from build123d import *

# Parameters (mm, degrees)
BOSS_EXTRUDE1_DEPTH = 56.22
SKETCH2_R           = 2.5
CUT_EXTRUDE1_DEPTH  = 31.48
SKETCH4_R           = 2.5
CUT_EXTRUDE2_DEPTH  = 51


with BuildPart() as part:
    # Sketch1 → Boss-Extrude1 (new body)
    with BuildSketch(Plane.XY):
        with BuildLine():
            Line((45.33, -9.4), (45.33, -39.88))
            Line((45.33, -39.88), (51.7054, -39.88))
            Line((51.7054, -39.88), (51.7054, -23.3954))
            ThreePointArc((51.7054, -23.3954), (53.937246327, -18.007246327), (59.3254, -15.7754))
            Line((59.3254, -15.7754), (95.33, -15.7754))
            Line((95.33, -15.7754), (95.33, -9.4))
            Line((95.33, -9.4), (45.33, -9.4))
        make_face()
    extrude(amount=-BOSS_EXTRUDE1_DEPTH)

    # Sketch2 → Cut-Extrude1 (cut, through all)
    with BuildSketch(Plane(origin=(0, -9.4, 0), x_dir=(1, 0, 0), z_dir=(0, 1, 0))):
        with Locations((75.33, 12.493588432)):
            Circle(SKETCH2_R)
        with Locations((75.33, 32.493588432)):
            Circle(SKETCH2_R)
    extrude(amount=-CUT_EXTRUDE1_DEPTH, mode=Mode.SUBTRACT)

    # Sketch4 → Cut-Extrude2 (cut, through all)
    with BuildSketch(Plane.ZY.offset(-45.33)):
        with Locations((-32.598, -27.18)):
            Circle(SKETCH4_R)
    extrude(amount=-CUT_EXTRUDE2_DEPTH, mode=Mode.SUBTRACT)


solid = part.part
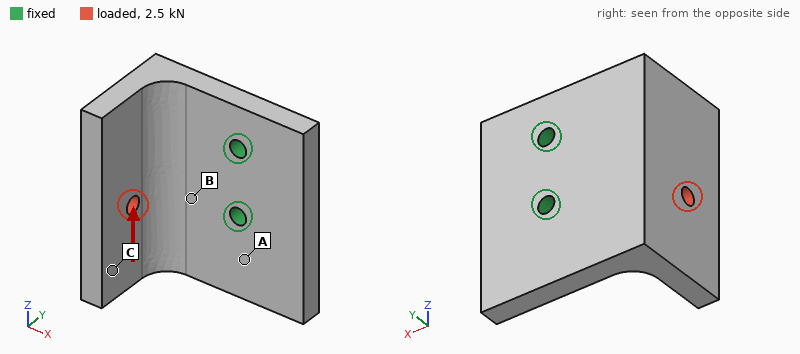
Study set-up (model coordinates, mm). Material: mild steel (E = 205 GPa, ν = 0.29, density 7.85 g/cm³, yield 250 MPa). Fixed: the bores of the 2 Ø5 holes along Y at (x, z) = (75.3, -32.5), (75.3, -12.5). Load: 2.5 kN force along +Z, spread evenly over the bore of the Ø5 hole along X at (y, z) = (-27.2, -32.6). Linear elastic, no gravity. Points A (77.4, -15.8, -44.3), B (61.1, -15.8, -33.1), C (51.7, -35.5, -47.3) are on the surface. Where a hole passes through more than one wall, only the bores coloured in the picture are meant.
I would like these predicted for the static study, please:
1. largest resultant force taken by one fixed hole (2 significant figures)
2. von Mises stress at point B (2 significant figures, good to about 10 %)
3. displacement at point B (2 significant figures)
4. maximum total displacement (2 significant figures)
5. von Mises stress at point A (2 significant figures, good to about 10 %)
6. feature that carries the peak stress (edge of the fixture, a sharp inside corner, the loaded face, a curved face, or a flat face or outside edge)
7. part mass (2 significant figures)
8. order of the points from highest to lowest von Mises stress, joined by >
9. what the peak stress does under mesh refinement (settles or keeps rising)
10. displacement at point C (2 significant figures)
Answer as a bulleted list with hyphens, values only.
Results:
- 3.4 kN
- 57 MPa
- 8.4 µm
- 56 µm
- 30 MPa
- edge of the fixture
- 210 g
- B > A > C
- keeps rising
- 44 µm
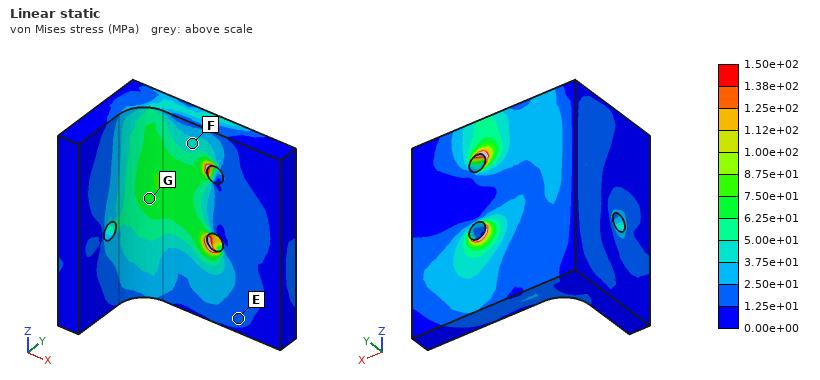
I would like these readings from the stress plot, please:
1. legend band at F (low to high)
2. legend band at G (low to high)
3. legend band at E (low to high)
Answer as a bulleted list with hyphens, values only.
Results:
- 3.75e+01 to 5.00e+01 MPa
- 6.25e+01 to 7.50e+01 MPa
- 1.25e+01 to 2.50e+01 MPa
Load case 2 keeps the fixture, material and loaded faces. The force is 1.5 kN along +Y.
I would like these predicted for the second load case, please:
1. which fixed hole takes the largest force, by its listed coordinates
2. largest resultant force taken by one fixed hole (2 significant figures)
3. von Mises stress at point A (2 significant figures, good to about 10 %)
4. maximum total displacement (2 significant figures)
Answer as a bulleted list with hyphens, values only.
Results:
- (75.3, -32.5)
- 1.2 kN
- 45 MPa
- 95 µm
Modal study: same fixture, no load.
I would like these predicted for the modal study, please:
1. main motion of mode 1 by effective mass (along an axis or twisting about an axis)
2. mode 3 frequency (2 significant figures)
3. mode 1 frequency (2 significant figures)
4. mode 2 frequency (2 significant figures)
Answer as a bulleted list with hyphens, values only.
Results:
- along Y
- 7500 Hz
- 2300 Hz
- 3800 Hz
